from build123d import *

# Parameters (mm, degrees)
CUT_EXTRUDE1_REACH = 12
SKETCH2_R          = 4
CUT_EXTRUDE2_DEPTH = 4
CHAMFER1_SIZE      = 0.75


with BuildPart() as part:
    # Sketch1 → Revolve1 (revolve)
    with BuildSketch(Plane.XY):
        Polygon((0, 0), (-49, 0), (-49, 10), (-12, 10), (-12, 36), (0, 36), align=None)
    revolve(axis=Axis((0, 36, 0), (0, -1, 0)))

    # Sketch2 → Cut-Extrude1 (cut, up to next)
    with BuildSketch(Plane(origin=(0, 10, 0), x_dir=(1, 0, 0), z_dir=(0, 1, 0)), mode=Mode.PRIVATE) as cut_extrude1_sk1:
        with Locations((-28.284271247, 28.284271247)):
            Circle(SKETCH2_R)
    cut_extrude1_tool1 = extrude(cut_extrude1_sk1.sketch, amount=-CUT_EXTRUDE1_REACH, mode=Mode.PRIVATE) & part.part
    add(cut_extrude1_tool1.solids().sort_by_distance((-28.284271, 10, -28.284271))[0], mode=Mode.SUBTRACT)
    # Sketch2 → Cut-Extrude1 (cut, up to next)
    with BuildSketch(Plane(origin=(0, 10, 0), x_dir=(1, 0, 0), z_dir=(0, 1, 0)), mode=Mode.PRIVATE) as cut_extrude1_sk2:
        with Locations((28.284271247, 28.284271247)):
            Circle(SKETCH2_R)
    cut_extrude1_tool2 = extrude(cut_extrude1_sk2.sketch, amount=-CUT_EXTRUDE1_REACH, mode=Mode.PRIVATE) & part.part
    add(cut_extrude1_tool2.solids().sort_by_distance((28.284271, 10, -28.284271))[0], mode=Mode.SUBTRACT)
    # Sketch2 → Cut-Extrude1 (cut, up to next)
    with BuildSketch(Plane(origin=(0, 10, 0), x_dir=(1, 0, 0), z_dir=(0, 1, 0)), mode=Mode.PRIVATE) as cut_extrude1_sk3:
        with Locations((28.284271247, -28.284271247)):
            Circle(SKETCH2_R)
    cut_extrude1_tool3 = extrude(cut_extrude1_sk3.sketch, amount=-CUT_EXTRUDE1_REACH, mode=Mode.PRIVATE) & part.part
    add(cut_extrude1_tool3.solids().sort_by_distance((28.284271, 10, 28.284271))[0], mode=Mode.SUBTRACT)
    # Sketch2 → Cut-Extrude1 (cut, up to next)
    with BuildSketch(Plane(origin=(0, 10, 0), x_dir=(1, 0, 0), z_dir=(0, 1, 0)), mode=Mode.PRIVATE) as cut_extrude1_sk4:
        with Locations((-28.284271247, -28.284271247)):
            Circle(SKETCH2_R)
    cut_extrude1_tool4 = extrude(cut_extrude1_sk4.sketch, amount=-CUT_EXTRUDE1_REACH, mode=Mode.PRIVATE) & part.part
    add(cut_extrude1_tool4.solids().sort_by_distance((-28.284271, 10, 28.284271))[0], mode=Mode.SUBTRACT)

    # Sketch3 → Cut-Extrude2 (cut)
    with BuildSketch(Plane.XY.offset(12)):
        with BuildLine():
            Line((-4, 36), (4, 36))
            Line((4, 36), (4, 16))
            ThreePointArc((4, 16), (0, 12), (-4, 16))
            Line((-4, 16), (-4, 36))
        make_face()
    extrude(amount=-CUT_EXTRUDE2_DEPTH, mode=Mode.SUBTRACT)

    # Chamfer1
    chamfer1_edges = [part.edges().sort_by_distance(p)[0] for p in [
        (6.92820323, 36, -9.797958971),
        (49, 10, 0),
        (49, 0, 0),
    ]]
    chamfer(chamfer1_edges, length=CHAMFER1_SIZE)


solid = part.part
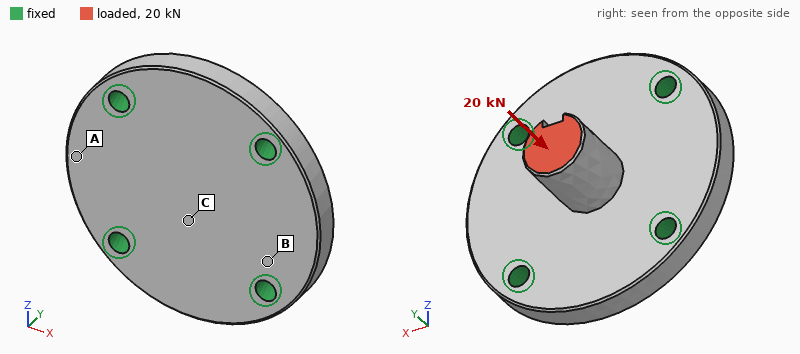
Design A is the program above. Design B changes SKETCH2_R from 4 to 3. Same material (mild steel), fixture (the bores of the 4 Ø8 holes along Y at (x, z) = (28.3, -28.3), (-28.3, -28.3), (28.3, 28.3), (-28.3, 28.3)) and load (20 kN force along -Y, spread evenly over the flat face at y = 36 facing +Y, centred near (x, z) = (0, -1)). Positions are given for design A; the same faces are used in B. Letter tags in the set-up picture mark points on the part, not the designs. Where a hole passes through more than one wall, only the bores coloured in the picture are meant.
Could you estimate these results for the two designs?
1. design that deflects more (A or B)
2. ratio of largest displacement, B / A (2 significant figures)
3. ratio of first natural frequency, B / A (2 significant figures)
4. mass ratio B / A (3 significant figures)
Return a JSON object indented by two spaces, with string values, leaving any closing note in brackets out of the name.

{
  "design that deflects more": "B",
  "ratio of largest displacement, B / A": "1.1",
  "ratio of first natural frequency, B / A": "0.93",
  "mass ratio B / A": "1.01"
}
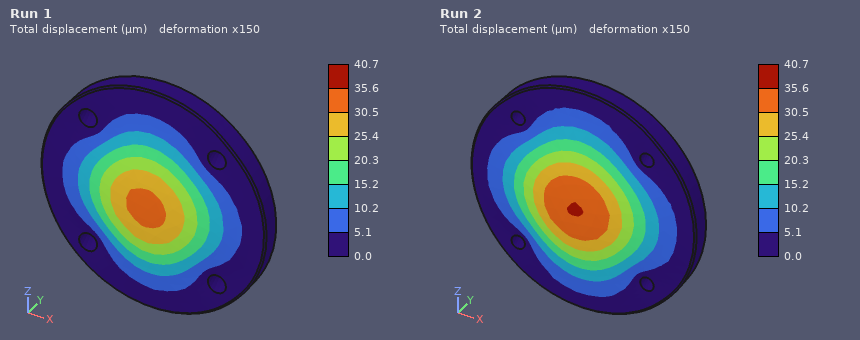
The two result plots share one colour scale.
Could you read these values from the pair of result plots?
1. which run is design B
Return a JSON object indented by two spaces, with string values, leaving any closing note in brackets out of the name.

{
  "which run is design B": "Run 2"
}
